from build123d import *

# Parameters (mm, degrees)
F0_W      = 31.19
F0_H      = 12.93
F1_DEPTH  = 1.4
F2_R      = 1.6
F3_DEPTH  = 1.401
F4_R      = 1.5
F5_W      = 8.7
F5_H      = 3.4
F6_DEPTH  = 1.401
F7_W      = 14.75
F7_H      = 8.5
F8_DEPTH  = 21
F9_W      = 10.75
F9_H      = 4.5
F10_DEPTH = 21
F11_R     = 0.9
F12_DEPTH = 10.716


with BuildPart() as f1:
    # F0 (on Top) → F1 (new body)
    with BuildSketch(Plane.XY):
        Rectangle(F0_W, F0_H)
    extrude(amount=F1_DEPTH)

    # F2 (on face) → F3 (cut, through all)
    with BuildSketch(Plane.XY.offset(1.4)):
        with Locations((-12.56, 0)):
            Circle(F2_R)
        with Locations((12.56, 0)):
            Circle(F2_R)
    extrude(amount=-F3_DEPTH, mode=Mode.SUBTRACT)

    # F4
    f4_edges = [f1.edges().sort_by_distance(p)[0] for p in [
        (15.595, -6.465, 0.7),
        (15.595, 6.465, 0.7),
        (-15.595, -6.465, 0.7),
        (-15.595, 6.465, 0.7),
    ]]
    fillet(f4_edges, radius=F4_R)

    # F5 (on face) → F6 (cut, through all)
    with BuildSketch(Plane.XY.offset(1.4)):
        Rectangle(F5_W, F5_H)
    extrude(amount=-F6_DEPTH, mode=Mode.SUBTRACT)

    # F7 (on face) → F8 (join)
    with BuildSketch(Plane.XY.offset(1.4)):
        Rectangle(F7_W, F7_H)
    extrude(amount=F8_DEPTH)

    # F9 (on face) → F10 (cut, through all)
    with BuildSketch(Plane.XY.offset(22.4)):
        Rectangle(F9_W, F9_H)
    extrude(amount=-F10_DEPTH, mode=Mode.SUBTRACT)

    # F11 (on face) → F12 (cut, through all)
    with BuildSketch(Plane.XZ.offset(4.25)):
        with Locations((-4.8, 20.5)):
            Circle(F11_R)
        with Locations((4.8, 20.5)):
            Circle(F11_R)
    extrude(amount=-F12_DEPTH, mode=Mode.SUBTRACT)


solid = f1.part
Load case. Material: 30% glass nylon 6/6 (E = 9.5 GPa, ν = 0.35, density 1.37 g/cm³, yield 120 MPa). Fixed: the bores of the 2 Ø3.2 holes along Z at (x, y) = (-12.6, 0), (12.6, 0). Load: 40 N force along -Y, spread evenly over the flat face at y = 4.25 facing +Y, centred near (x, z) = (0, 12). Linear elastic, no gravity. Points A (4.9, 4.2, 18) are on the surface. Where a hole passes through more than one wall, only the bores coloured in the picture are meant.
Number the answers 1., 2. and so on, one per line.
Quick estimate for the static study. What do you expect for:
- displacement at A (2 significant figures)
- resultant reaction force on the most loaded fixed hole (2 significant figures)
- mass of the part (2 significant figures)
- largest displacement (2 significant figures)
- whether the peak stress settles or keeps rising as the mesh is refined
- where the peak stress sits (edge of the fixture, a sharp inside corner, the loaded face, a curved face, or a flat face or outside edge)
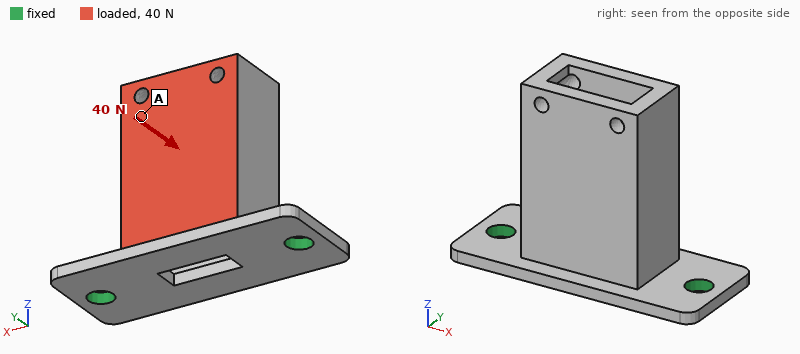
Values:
1. 0.32 mm
2. 20 N
3. 2.9 g
4. 0.40 mm
5. keeps rising
6. edge of the fixture
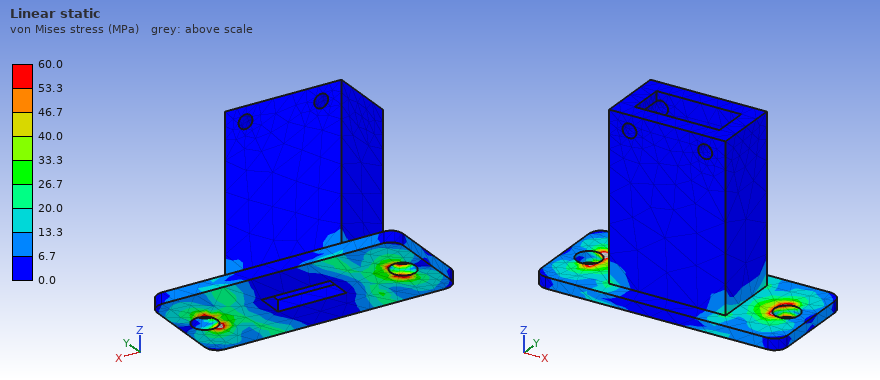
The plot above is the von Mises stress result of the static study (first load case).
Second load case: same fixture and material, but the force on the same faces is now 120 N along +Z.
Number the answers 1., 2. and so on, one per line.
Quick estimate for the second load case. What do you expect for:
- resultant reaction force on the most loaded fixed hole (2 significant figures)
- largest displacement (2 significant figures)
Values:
1. 67 N
2. 0.46 mm
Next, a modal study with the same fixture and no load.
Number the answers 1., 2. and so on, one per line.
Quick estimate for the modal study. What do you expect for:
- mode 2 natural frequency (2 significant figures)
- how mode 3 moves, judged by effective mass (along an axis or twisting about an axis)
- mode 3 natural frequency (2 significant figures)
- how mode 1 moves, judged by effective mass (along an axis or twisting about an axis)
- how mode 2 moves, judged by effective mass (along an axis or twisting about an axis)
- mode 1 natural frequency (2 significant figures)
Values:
1. 4000 Hz
2. along Z
3. 5500 Hz
4. along Y
5. along X
6. 1300 Hz
